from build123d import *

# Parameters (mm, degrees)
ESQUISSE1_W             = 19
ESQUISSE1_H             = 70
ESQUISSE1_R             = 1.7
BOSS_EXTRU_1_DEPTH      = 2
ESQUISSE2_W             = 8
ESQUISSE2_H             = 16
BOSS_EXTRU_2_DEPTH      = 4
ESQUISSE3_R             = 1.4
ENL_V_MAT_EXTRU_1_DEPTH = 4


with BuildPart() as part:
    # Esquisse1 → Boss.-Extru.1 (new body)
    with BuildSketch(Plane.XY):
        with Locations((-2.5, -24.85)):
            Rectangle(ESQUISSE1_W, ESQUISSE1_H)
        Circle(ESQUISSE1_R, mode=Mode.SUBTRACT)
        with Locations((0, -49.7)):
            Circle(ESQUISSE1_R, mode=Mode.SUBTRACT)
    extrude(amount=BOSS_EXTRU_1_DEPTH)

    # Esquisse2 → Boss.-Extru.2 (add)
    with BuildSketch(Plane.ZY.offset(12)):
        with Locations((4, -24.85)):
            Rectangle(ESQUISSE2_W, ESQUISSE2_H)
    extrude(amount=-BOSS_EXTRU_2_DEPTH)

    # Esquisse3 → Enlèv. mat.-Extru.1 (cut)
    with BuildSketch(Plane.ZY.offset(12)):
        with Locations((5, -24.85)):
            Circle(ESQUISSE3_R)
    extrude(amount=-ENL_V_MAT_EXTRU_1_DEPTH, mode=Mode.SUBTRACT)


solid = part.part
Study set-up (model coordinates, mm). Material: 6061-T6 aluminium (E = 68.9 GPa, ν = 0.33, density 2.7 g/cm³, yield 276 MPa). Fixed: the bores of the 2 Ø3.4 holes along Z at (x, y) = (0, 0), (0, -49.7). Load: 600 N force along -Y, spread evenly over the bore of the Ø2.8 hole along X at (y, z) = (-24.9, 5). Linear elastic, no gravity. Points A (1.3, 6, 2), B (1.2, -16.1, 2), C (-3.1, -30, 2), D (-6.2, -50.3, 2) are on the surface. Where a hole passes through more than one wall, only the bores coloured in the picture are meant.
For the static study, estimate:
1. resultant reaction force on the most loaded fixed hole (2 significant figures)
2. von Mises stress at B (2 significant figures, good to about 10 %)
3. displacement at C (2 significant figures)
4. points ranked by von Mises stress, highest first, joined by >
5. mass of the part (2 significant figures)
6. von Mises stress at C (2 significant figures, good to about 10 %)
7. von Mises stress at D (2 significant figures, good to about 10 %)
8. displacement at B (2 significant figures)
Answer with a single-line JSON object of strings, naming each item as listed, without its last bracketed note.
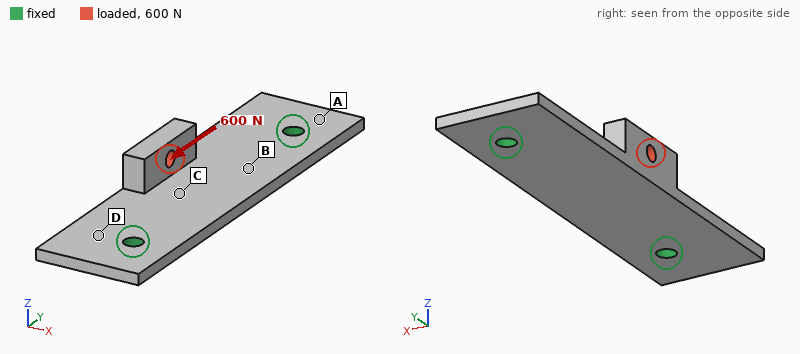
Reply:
{"resultant reaction force on the most loaded fixed hole": "330 N", "von Mises stress at B": "30 MPa", "displacement at C": "18 µm", "points ranked by von Mises stress, highest first, joined by >": "C > B > D > A", "mass of the part": "8.1 g", "von Mises stress at C": "43 MPa", "von Mises stress at D": "19 MPa", "displacement at B": "15 µm"}
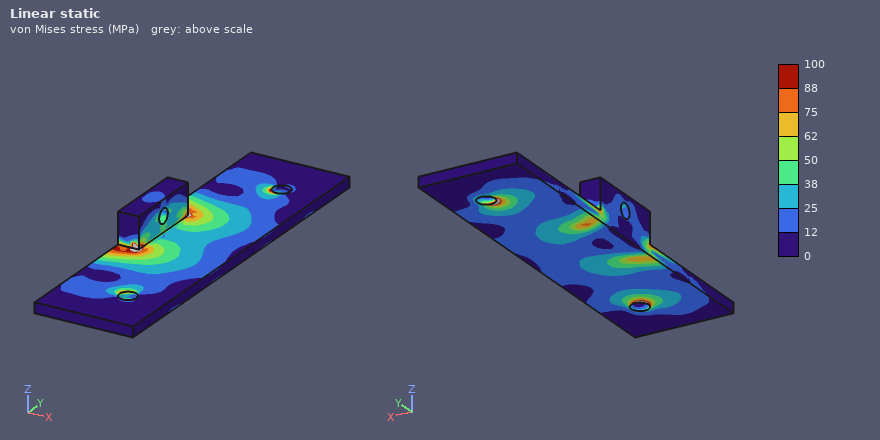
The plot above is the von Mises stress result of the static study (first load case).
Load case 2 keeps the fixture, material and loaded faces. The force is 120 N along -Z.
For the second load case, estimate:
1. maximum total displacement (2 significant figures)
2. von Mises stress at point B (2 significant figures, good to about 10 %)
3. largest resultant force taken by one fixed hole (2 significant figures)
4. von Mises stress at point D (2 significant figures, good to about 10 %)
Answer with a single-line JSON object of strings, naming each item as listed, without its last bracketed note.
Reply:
{"maximum total displacement": "0.12 mm", "von Mises stress at point B": "20 MPa", "largest resultant force taken by one fixed hole": "62 N", "von Mises stress at point D": "37 MPa"}
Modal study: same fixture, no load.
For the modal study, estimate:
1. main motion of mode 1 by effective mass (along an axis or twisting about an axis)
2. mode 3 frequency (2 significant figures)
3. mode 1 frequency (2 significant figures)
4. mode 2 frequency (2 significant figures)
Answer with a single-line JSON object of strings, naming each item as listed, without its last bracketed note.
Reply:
{"main motion of mode 1 by effective mass": "along Z", "mode 3 frequency": "9300 Hz", "mode 1 frequency": "3700 Hz", "mode 2 frequency": "5700 Hz"}
